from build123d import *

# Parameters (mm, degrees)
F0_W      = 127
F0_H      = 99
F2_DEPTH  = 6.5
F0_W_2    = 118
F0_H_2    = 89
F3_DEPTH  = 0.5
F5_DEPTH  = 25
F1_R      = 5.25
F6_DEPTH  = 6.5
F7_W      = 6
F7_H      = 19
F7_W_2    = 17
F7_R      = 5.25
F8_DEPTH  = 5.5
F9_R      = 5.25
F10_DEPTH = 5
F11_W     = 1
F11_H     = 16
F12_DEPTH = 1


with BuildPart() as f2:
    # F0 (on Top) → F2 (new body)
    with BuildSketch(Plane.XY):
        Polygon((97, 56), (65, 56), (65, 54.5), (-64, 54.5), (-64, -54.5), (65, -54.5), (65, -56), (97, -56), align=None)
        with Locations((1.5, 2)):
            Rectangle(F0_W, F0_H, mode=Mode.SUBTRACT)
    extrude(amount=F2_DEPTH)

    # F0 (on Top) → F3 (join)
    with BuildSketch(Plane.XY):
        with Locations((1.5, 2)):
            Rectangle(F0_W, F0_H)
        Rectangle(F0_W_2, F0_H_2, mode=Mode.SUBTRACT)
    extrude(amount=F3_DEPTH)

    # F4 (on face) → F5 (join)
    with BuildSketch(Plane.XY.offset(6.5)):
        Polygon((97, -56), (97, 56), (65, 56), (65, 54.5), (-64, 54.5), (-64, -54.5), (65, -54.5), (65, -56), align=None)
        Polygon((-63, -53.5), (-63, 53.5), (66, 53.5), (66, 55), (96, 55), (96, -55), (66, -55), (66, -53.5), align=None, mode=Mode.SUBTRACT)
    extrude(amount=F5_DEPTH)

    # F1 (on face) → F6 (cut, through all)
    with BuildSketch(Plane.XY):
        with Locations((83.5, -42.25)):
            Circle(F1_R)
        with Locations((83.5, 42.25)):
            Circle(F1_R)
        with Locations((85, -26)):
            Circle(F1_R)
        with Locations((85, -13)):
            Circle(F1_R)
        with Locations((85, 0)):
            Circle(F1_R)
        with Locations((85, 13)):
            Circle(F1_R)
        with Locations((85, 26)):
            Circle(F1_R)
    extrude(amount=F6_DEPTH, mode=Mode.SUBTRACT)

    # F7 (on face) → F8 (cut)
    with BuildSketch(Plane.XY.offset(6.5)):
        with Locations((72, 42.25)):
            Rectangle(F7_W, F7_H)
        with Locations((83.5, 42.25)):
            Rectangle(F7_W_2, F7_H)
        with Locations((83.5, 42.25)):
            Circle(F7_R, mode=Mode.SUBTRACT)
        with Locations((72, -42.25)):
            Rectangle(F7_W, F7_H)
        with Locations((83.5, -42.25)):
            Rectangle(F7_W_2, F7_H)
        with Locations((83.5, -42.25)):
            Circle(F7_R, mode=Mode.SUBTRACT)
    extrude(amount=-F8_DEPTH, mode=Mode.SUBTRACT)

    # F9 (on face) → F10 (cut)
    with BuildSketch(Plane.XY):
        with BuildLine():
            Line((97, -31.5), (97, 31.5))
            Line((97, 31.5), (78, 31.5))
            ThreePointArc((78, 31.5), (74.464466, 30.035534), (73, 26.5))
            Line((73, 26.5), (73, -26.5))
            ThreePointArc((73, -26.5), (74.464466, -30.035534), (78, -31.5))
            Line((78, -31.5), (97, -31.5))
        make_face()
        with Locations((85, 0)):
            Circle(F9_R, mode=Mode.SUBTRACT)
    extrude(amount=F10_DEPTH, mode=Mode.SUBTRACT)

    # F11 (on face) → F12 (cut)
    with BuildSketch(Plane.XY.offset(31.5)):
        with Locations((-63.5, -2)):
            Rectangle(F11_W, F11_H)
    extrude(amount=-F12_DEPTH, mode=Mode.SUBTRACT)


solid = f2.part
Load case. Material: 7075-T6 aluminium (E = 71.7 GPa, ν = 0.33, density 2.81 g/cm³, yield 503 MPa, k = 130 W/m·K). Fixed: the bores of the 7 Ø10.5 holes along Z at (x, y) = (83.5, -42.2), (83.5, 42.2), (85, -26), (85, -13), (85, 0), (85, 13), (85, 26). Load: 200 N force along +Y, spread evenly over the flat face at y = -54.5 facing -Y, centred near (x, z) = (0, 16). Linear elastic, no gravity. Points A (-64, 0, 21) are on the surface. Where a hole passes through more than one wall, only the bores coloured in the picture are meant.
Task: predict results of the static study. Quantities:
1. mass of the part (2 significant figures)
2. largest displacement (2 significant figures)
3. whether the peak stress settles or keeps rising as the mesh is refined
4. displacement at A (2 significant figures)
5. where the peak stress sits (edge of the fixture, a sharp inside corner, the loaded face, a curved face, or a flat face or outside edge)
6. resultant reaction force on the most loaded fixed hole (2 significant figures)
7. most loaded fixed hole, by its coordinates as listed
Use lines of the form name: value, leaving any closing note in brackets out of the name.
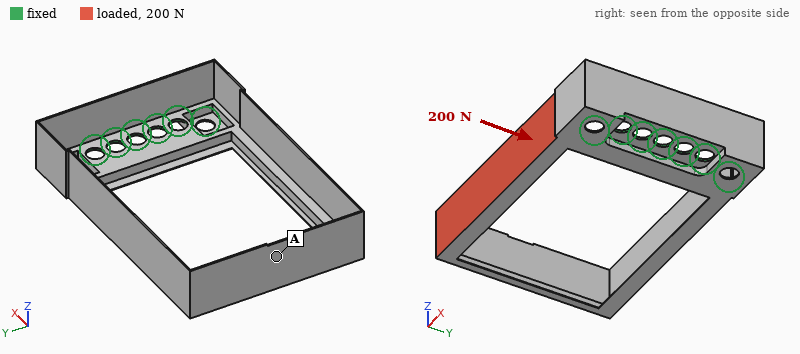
mass of the part: 97 g
largest displacement: 1.9 mm
whether the peak stress settles or keeps rising as the mesh is refined: keeps rising
displacement at A: 1.8 mm
where the peak stress sits: a sharp inside corner
resultant reaction force on the most loaded fixed hole: 320 N
most loaded fixed hole, by its coordinates as listed: (83.5, -42.2)
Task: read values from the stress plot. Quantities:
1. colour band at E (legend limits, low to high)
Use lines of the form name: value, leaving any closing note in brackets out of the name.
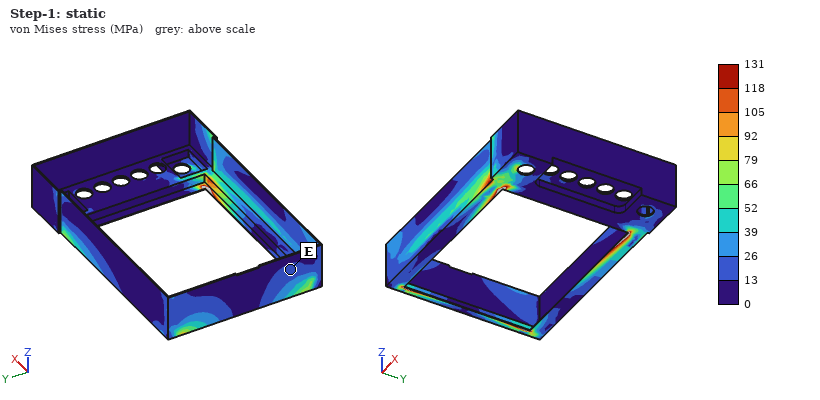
colour band at E: 13 to 26 MPa
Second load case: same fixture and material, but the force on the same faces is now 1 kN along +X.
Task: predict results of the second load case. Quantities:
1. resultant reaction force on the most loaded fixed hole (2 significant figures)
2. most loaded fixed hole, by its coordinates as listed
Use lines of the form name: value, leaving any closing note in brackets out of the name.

resultant reaction force on the most loaded fixed hole: 1.2 kN
most loaded fixed hole, by its coordinates as listed: (85, -26)
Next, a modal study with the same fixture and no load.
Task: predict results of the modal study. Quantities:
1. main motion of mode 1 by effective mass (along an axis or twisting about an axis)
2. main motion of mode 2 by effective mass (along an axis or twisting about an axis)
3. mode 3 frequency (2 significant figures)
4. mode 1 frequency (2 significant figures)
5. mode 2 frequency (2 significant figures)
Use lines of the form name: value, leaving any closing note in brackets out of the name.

main motion of mode 1 by effective mass: along Y
main motion of mode 2 by effective mass: along Z
mode 3 frequency: 360 Hz
mode 1 frequency: 230 Hz
mode 2 frequency: 270 Hz
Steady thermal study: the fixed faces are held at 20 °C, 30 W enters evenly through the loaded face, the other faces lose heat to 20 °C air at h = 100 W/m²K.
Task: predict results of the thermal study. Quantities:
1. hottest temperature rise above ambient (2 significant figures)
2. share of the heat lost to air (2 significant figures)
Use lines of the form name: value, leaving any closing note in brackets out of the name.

hottest temperature rise above ambient: 38 K
share of the heat lost to air: 87 %
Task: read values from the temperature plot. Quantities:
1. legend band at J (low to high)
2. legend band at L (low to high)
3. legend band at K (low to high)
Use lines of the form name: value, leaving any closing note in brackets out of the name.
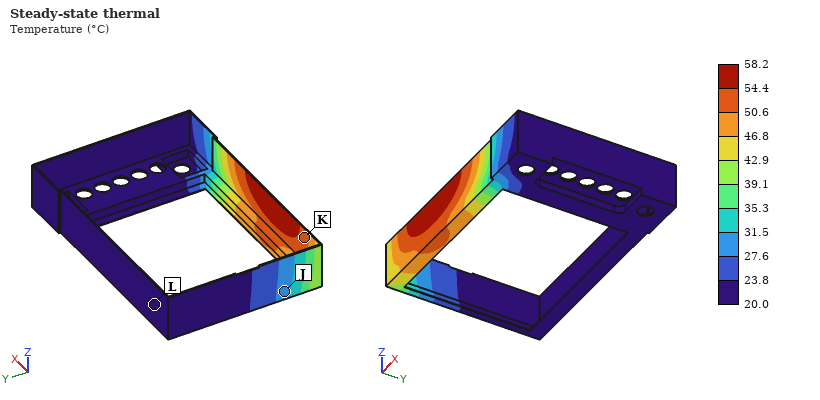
legend band at J: 27.6 to 31.5 °C
legend band at L: 20.0 to 23.8 °C
legend band at K: 50.6 to 54.4 °C
